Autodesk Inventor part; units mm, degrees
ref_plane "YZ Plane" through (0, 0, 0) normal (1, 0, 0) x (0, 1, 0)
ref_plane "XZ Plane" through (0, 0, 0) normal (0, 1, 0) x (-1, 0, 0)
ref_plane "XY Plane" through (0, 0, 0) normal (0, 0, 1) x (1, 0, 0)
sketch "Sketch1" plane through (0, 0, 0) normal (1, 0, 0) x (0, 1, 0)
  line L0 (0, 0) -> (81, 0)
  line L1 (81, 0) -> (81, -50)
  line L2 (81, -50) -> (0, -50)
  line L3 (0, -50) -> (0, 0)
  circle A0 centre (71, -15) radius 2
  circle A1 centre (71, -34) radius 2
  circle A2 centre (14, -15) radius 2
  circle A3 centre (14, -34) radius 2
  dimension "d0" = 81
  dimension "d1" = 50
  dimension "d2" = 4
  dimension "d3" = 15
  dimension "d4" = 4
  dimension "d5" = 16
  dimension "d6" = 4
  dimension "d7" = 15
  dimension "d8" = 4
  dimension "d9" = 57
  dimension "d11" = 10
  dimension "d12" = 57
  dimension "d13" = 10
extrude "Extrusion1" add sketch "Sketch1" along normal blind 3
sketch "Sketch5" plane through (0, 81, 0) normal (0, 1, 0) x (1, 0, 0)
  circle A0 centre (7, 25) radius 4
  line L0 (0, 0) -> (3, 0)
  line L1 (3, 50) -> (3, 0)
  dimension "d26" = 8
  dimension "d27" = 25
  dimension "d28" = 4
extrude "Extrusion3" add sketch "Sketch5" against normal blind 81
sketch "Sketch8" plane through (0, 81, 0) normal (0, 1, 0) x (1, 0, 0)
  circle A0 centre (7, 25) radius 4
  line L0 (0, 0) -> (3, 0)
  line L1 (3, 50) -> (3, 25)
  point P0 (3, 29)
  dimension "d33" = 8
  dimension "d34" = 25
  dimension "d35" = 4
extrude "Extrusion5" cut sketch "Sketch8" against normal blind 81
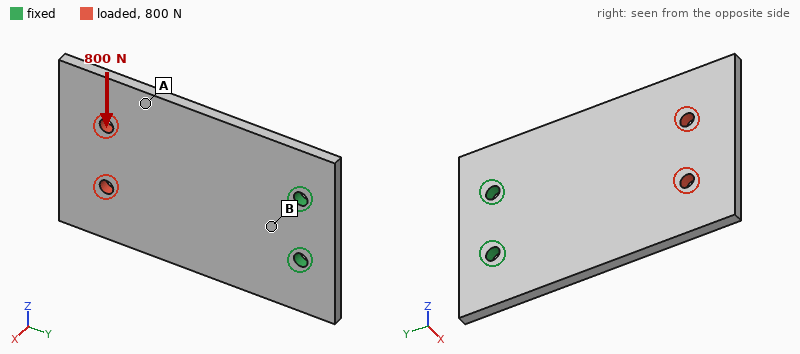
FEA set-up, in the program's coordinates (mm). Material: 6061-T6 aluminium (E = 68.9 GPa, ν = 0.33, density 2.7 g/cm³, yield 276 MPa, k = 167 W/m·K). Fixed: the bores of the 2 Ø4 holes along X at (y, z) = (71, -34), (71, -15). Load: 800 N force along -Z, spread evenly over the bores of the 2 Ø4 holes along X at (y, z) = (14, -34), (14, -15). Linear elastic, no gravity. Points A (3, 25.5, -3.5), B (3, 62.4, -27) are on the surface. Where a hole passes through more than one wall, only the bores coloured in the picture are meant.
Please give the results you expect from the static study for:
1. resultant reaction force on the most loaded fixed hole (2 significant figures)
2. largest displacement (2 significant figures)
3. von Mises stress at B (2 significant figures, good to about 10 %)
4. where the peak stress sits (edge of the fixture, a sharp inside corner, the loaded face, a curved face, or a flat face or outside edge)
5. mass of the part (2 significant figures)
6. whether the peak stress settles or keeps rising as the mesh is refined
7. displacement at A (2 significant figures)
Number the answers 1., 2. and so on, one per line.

1. 2.1 kN
2. 95 µm
3. 33 MPa
4. edge of the fixture
5. 32 g
6. keeps rising
7. 61 µm
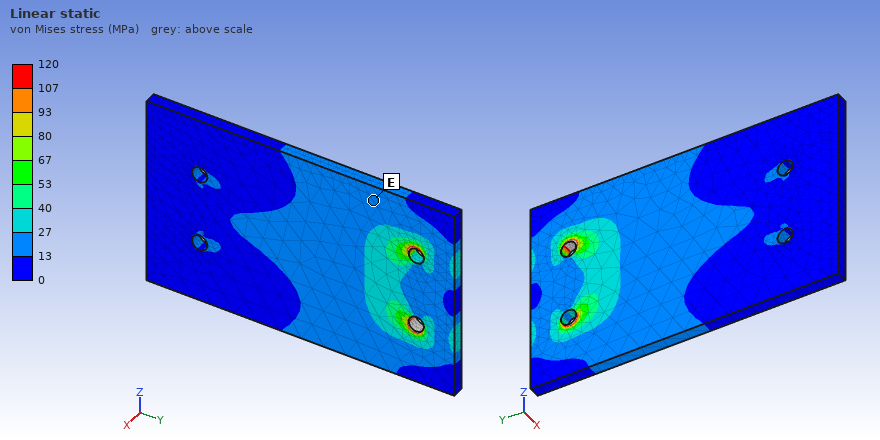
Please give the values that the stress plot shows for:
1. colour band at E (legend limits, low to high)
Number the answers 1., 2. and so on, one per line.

1. 13 to 27 MPa
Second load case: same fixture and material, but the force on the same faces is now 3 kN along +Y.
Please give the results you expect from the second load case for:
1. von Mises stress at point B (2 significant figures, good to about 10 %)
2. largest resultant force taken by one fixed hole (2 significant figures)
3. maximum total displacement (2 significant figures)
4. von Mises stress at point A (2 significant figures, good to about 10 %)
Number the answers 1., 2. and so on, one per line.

1. 21 MPa
2. 1.5 kN
3. 24 µm
4. 15 MPa
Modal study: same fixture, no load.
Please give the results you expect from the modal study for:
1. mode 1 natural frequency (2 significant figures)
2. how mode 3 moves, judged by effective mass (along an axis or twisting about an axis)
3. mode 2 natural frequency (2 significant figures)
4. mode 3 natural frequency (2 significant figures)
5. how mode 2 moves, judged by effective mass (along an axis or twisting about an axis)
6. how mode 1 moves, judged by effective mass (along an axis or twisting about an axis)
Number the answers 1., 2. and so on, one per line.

1. 490 Hz
2. along X
3. 1500 Hz
4. 3000 Hz
5. twisting about Y
6. along X
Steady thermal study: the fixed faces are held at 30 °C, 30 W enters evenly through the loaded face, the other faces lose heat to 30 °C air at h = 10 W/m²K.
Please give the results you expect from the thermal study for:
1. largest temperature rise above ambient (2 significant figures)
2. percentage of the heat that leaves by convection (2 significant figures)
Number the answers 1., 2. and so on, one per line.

1. 72 K
2. 10 %
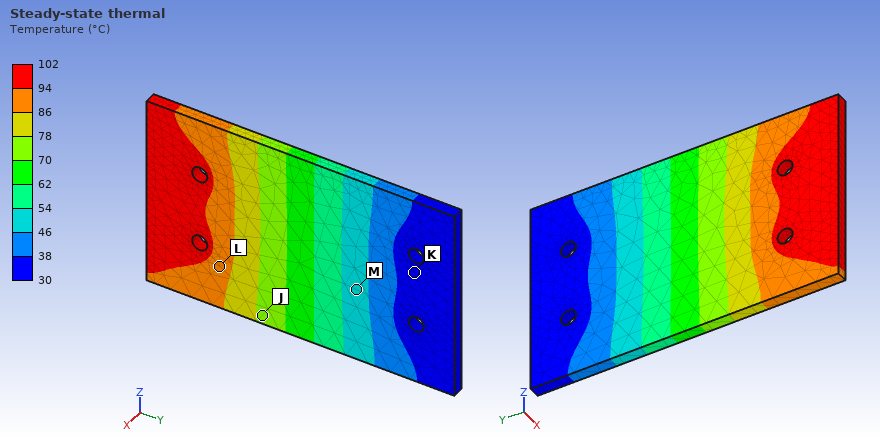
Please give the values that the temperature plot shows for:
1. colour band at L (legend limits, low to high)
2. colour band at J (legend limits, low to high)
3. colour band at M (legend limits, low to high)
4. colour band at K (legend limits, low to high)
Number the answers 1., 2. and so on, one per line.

1. 86 to 94 °C
2. 70 to 78 °C
3. 46 to 54 °C
4. 30 to 38 °C
